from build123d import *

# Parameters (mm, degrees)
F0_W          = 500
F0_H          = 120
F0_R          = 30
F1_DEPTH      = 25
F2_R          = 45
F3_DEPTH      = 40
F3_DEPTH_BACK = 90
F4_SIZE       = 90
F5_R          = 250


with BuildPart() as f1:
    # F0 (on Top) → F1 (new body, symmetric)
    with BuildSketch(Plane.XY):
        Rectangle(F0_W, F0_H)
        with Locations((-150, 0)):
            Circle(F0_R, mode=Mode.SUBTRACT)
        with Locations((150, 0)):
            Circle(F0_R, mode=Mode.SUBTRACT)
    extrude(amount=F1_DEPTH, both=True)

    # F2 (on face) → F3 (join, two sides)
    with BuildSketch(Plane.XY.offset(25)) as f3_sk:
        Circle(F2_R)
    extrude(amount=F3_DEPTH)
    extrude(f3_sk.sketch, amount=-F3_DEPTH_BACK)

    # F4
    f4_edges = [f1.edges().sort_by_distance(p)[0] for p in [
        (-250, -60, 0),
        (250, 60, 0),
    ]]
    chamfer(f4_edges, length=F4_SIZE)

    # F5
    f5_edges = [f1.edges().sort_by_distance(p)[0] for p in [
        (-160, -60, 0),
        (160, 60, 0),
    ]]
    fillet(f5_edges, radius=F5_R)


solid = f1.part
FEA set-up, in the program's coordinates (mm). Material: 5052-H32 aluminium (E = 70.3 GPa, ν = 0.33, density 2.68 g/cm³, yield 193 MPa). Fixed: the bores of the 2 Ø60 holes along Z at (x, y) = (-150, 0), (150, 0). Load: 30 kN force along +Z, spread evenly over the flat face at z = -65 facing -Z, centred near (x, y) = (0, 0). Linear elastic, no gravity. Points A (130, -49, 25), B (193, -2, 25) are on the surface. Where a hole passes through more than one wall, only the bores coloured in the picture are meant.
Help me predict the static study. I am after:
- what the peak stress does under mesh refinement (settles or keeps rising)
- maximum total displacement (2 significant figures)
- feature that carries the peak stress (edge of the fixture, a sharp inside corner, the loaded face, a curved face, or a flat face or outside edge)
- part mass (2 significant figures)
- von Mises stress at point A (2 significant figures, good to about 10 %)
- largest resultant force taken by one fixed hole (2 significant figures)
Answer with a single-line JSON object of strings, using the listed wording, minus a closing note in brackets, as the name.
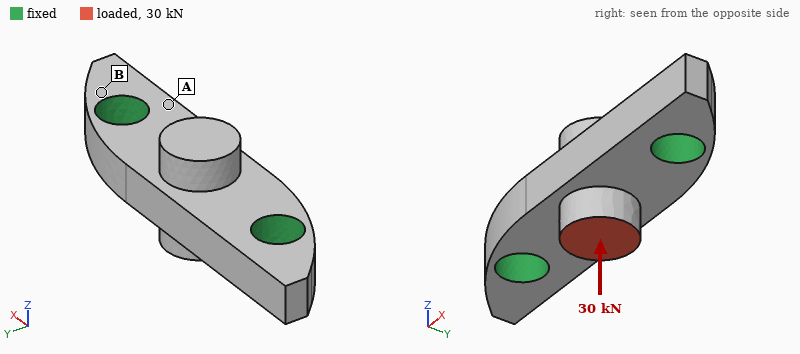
{"what the peak stress does under mesh refinement": "keeps rising", "maximum total displacement": "31 µm", "feature that carries the peak stress": "edge of the fixture", "part mass": "7.2 kg", "von Mises stress at point A": "6.5 MPa", "largest resultant force taken by one fixed hole": "15 kN"}
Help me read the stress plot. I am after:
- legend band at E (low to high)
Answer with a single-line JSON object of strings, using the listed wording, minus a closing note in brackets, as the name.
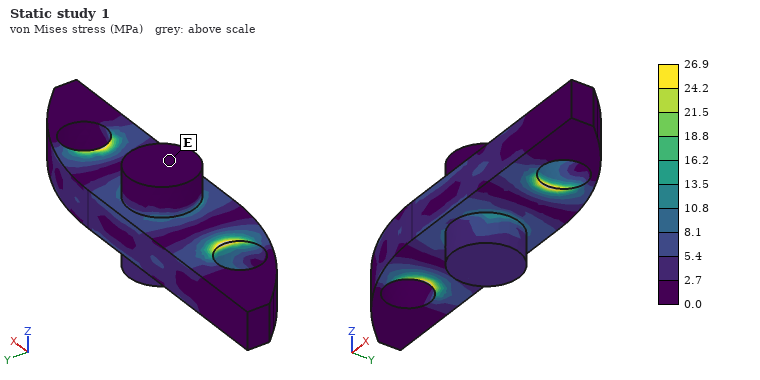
{"legend band at E": "0.0 to 2.7 MPa"}
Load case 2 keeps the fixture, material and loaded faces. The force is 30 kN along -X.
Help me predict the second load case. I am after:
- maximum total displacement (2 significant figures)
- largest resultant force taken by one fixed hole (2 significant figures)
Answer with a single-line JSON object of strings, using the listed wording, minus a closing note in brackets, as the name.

{"maximum total displacement": "37 µm", "largest resultant force taken by one fixed hole": "18 kN"}
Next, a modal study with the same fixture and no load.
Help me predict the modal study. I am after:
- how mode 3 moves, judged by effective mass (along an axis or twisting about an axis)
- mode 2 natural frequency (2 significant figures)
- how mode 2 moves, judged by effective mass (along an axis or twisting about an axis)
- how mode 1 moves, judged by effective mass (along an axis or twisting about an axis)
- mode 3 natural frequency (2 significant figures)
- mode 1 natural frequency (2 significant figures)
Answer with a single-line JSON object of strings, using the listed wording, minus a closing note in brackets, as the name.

{"how mode 3 moves, judged by effective mass": "along Y", "mode 2 natural frequency": "2900 Hz", "how mode 2 moves, judged by effective mass": "twisting about X", "how mode 1 moves, judged by effective mass": "along Z", "mode 3 natural frequency": "3300 Hz", "mode 1 natural frequency": "2800 Hz"}
